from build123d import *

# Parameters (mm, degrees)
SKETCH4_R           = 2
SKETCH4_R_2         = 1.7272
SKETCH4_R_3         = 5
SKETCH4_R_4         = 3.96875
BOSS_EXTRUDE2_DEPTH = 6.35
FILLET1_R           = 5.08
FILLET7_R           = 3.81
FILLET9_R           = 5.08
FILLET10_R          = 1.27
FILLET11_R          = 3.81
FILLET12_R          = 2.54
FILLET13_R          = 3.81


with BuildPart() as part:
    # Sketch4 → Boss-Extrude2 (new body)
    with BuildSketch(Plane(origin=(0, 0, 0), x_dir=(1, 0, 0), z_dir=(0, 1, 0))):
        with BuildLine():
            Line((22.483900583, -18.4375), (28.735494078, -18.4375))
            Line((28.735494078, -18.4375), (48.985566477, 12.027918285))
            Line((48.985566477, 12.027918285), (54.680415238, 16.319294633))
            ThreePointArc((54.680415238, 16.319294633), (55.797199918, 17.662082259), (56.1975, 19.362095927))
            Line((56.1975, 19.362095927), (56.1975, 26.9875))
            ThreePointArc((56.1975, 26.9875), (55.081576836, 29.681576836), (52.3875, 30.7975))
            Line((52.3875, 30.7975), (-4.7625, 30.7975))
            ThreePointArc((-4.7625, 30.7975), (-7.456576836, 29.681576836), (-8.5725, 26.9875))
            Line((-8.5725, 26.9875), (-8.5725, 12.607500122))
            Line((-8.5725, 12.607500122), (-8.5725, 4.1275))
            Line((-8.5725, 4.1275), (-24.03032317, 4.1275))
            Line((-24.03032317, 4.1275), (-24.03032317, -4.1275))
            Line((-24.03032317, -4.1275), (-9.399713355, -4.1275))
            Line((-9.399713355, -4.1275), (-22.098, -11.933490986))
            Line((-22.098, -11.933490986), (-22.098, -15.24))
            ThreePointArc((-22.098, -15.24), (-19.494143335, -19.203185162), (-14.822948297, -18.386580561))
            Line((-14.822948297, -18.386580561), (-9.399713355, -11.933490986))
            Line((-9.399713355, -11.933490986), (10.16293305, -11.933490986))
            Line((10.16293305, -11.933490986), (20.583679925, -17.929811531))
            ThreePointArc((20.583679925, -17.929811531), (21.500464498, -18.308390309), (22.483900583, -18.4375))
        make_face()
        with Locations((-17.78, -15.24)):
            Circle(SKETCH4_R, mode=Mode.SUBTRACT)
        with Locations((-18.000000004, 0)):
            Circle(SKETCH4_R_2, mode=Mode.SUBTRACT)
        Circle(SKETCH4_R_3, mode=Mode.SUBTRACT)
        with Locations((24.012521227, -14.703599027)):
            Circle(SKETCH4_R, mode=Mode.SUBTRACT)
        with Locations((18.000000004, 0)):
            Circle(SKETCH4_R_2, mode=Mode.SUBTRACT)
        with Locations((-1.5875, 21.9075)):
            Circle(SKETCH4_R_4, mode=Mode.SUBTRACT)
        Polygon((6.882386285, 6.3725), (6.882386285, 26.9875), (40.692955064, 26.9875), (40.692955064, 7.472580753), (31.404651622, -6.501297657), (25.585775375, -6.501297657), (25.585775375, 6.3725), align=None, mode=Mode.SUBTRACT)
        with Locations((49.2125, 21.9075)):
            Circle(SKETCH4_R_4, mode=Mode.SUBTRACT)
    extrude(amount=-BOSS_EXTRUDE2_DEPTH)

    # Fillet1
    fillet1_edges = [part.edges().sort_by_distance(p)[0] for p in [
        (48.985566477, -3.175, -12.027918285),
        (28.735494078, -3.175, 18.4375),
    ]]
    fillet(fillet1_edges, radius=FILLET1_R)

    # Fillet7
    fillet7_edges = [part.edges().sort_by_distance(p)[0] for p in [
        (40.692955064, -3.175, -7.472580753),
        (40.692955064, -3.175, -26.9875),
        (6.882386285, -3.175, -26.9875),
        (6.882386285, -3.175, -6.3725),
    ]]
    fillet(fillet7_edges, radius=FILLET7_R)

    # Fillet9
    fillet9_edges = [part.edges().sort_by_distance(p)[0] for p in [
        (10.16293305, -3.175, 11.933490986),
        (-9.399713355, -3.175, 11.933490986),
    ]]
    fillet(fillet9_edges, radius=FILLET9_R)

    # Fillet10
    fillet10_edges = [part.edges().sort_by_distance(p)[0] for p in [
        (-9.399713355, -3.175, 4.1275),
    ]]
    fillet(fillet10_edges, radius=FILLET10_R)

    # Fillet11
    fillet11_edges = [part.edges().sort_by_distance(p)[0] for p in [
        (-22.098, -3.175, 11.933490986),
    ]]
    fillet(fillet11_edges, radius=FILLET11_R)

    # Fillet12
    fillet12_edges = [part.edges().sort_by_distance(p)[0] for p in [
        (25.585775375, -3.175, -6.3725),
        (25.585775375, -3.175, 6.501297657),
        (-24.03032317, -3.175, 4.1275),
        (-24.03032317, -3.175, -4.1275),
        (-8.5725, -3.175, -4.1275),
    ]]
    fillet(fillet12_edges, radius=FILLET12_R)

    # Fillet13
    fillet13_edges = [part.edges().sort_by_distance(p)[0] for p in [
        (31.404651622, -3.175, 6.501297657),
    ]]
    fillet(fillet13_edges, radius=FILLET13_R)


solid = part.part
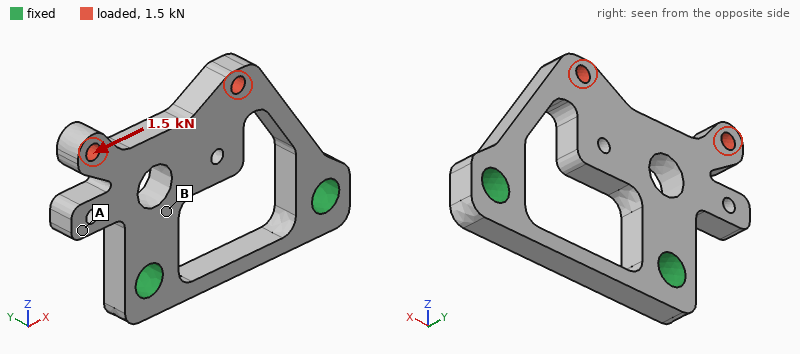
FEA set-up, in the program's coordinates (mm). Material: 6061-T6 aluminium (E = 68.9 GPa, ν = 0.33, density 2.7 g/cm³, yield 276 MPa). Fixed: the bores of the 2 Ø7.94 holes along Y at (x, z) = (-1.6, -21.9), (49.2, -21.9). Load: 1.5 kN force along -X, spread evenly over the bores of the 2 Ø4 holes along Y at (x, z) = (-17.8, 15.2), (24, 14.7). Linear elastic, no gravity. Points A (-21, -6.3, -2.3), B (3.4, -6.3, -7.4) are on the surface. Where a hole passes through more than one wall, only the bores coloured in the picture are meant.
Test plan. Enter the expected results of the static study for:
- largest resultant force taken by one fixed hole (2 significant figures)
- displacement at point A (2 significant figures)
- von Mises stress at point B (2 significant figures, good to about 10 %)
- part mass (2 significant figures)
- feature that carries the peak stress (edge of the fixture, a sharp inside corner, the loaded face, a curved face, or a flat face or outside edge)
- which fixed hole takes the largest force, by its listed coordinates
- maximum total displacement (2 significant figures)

1.2 kN
31 µm
30 MPa
29 g
a curved face
(-1.6, -21.9)
90 µm
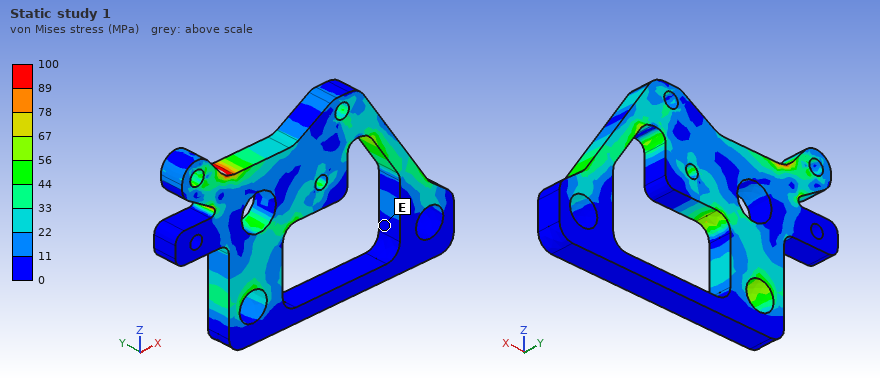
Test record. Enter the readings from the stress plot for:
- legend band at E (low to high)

0 to 11 MPa
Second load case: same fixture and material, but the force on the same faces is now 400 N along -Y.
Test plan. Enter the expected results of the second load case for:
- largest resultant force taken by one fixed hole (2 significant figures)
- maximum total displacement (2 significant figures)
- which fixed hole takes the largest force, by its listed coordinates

320 N
0.28 mm
(-1.6, -21.9)
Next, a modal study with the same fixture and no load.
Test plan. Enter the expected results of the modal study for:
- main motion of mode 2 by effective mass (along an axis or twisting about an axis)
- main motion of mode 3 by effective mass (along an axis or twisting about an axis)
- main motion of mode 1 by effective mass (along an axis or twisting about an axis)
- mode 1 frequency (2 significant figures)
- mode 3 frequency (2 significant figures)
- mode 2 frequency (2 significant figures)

twisting about Z
along X
along Y
2800 Hz
9200 Hz
4200 Hz
